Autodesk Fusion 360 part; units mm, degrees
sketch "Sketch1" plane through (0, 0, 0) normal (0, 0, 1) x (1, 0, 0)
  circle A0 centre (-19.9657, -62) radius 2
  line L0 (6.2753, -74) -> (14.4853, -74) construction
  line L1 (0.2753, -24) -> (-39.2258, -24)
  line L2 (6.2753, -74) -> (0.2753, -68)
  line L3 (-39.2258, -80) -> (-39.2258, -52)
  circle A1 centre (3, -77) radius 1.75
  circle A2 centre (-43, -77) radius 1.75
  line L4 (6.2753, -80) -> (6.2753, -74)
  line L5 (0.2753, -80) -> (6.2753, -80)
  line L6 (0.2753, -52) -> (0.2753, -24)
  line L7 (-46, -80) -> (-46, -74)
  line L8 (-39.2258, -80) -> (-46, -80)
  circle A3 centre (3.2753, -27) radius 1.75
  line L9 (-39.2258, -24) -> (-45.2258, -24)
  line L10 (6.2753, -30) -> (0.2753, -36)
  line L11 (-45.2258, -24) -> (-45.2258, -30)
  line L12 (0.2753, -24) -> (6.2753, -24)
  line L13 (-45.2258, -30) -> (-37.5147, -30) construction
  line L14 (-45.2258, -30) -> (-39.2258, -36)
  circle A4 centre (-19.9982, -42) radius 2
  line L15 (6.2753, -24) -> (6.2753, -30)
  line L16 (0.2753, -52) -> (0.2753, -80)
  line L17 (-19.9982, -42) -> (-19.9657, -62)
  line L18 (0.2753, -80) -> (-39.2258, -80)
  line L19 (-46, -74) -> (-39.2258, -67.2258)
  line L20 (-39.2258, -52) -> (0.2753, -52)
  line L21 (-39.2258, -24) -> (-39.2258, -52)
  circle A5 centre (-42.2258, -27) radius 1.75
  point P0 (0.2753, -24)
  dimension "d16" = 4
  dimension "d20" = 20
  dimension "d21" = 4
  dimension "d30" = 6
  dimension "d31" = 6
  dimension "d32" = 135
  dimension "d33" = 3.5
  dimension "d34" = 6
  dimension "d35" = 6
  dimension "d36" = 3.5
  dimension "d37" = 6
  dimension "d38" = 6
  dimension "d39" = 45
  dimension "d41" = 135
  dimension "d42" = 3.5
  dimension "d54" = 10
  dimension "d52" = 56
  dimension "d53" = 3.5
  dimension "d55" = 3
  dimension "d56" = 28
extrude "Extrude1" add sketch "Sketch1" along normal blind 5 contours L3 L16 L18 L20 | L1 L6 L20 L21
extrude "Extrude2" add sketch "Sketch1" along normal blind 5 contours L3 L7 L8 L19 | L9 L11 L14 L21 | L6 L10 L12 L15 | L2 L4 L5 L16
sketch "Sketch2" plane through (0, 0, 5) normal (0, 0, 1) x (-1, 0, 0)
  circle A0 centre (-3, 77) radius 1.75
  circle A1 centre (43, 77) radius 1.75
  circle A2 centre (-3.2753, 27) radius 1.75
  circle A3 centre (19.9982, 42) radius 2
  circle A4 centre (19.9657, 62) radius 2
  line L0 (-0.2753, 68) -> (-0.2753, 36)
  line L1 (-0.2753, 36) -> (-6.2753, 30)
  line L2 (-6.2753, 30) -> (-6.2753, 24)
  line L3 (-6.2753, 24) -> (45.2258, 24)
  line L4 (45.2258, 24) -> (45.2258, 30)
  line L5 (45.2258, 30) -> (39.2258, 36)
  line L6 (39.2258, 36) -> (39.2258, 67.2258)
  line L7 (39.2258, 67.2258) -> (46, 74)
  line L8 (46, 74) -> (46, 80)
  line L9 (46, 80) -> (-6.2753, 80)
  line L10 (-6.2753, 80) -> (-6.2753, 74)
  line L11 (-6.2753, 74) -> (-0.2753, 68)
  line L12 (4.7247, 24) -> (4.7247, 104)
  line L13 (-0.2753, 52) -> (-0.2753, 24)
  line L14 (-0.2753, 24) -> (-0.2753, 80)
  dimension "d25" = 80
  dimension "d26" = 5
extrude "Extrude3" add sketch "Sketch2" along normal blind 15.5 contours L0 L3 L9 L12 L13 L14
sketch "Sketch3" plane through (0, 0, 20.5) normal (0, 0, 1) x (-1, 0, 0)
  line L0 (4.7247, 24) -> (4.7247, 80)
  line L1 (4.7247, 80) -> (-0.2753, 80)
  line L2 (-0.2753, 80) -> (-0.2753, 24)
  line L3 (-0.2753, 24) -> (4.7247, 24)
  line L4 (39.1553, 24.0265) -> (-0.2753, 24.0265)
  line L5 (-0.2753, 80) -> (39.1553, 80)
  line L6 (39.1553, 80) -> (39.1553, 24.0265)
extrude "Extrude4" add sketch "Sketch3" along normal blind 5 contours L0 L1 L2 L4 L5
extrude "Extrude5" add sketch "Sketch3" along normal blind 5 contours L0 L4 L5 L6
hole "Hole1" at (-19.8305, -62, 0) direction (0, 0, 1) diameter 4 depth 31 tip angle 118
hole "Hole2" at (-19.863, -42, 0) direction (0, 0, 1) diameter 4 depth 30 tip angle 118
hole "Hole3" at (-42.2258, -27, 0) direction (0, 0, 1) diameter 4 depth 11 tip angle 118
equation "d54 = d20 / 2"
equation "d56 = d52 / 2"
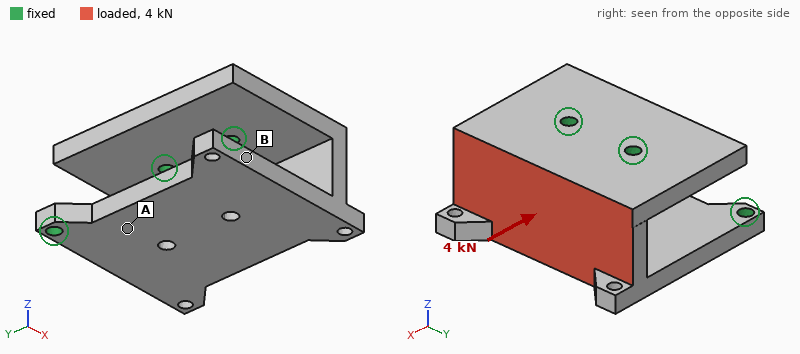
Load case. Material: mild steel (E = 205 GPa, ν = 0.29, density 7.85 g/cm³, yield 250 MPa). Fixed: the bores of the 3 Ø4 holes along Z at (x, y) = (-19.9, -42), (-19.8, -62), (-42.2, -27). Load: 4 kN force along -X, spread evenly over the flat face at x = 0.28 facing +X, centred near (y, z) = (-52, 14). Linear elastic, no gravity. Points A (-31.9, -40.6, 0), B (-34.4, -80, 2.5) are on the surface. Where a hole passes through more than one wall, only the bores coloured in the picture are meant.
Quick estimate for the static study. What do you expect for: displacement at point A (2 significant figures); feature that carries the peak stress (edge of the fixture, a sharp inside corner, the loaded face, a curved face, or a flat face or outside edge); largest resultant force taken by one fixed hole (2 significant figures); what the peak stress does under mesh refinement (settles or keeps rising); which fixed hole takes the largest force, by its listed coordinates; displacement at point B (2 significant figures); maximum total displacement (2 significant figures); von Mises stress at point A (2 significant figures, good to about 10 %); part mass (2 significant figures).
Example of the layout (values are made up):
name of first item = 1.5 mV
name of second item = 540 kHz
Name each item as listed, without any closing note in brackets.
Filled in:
displacement at point A = 7.2 µm
feature that carries the peak stress = edge of the fixture
largest resultant force taken by one fixed hole = 2.3 kN
what the peak stress does under mesh refinement = keeps rising
which fixed hole takes the largest force, by its listed coordinates = (-19.8, -62)
displacement at point B = 24 µm
maximum total displacement = 27 µm
von Mises stress at point A = 16 MPa
part mass = 210 g
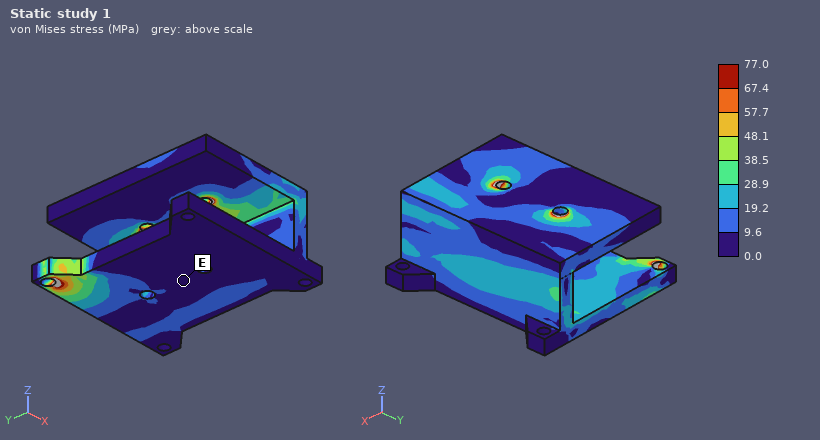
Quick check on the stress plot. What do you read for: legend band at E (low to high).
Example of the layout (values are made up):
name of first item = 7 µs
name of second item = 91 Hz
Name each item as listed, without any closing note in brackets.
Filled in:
legend band at E = 0.0 to 9.6 MPa
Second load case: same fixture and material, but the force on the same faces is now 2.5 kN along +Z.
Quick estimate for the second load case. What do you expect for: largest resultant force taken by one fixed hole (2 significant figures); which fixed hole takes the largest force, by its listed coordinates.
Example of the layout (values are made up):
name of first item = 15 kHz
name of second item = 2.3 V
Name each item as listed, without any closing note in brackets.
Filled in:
largest resultant force taken by one fixed hole = 2.1 kN
which fixed hole takes the largest force, by its listed coordinates = (-19.9, -42)
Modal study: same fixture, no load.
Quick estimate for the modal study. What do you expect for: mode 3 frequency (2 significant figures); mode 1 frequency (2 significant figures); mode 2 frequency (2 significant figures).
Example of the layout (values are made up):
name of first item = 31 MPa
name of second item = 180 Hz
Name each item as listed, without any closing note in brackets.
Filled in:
mode 3 frequency = 6200 Hz
mode 1 frequency = 2600 Hz
mode 2 frequency = 4300 Hz
